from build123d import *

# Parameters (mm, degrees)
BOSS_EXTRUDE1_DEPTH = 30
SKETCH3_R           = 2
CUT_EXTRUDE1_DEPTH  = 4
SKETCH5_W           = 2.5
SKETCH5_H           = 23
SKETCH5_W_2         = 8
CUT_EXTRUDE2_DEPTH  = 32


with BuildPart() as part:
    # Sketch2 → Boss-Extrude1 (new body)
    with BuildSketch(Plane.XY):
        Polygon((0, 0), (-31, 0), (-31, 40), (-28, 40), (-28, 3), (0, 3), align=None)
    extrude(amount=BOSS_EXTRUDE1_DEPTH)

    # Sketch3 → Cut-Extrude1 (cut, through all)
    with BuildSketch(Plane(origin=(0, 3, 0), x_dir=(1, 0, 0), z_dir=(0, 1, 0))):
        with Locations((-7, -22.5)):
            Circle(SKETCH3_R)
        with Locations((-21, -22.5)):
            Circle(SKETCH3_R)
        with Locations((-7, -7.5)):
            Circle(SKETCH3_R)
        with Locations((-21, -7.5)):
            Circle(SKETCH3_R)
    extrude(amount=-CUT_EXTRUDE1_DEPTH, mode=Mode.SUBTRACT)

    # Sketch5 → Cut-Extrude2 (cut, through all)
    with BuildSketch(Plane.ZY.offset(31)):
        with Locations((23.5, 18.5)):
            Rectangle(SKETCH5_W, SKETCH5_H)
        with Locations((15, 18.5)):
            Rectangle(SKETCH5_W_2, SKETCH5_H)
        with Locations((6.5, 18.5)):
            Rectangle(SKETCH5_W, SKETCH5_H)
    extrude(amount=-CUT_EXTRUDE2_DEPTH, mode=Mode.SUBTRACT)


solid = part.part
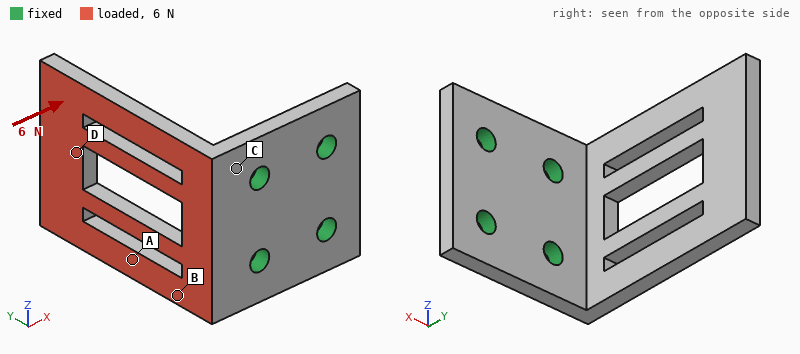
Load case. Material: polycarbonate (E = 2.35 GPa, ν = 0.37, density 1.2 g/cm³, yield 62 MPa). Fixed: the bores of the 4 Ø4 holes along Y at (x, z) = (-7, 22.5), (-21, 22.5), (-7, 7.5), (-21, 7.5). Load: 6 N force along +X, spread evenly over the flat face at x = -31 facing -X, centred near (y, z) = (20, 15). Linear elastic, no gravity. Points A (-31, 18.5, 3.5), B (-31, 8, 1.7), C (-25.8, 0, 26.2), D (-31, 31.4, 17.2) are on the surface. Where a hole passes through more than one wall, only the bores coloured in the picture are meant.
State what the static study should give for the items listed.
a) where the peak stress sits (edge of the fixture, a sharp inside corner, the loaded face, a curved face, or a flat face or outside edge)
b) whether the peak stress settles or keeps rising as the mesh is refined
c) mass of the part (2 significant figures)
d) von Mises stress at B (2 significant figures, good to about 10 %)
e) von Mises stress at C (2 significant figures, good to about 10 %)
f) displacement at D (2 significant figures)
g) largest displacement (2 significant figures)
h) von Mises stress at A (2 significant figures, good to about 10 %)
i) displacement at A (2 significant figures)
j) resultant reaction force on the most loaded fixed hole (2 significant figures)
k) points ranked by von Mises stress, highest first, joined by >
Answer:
edge of the fixture
keeps rising
6.1 g
2.8 MPa
2.2 MPa
0.43 mm
0.60 mm
1.5 MPa
0.19 mm
2.8 N
B > C > A > D
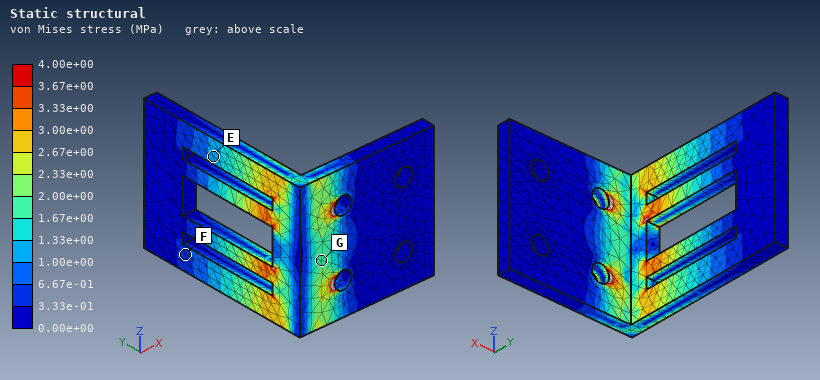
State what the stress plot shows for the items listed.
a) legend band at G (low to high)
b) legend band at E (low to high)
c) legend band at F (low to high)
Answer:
1.67e+00 to 2.00e+00 MPa
1.00e+00 to 1.33e+00 MPa
3.33e-01 to 6.67e-01 MPa
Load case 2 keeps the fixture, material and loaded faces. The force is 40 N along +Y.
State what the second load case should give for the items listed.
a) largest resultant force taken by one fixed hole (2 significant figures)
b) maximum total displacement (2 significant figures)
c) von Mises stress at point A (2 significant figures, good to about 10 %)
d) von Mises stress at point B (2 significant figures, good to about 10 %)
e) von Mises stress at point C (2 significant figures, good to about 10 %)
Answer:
22 N
0.65 mm
1.6 MPa
1.9 MPa
3.9 MPa
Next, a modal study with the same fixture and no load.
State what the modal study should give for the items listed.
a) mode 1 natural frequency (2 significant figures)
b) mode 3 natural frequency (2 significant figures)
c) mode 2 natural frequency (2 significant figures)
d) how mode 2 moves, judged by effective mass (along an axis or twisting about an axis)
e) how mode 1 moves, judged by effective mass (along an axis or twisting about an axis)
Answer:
340 Hz
1000 Hz
820 Hz
along Z
along X
